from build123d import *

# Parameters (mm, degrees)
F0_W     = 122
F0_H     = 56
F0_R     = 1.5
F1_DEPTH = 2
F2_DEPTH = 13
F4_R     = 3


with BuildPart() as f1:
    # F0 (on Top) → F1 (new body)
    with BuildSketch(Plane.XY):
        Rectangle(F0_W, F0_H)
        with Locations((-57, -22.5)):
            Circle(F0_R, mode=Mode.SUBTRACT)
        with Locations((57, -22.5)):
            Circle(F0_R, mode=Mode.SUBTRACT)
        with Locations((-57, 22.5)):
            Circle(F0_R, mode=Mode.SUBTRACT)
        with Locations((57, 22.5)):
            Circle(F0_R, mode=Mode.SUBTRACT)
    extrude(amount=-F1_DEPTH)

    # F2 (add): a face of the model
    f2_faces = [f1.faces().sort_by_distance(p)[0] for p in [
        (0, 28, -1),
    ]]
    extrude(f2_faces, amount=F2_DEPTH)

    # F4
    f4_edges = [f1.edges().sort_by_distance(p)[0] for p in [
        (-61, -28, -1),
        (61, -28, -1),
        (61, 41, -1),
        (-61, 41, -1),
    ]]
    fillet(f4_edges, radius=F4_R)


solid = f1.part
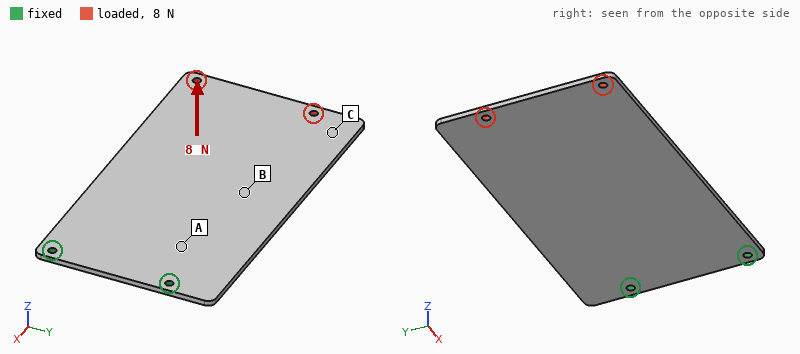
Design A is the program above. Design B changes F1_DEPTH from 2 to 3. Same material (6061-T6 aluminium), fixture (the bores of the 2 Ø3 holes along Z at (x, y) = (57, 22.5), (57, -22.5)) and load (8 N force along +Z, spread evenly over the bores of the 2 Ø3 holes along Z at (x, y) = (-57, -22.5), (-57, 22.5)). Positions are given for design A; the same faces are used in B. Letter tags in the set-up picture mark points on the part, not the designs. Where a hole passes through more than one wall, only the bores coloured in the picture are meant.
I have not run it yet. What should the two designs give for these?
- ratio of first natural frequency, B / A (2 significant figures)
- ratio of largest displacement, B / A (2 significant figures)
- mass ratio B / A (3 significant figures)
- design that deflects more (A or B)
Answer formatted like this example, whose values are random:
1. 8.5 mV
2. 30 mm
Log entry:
1. 1.5
2. 0.30
3. 1.50
4. A
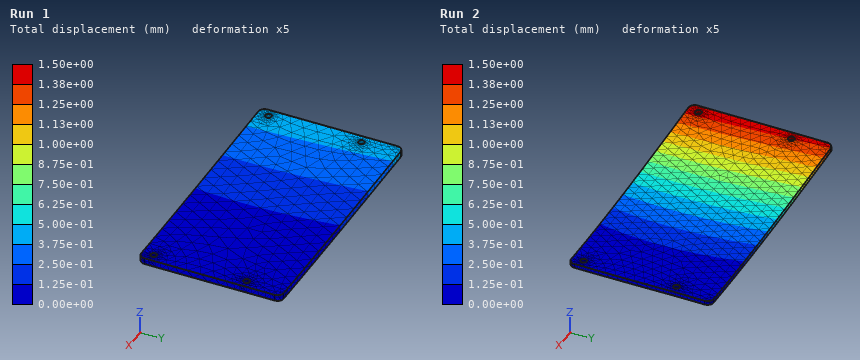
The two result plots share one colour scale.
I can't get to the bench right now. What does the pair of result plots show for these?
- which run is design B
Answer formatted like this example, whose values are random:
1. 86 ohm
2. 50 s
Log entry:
1. Run 1
